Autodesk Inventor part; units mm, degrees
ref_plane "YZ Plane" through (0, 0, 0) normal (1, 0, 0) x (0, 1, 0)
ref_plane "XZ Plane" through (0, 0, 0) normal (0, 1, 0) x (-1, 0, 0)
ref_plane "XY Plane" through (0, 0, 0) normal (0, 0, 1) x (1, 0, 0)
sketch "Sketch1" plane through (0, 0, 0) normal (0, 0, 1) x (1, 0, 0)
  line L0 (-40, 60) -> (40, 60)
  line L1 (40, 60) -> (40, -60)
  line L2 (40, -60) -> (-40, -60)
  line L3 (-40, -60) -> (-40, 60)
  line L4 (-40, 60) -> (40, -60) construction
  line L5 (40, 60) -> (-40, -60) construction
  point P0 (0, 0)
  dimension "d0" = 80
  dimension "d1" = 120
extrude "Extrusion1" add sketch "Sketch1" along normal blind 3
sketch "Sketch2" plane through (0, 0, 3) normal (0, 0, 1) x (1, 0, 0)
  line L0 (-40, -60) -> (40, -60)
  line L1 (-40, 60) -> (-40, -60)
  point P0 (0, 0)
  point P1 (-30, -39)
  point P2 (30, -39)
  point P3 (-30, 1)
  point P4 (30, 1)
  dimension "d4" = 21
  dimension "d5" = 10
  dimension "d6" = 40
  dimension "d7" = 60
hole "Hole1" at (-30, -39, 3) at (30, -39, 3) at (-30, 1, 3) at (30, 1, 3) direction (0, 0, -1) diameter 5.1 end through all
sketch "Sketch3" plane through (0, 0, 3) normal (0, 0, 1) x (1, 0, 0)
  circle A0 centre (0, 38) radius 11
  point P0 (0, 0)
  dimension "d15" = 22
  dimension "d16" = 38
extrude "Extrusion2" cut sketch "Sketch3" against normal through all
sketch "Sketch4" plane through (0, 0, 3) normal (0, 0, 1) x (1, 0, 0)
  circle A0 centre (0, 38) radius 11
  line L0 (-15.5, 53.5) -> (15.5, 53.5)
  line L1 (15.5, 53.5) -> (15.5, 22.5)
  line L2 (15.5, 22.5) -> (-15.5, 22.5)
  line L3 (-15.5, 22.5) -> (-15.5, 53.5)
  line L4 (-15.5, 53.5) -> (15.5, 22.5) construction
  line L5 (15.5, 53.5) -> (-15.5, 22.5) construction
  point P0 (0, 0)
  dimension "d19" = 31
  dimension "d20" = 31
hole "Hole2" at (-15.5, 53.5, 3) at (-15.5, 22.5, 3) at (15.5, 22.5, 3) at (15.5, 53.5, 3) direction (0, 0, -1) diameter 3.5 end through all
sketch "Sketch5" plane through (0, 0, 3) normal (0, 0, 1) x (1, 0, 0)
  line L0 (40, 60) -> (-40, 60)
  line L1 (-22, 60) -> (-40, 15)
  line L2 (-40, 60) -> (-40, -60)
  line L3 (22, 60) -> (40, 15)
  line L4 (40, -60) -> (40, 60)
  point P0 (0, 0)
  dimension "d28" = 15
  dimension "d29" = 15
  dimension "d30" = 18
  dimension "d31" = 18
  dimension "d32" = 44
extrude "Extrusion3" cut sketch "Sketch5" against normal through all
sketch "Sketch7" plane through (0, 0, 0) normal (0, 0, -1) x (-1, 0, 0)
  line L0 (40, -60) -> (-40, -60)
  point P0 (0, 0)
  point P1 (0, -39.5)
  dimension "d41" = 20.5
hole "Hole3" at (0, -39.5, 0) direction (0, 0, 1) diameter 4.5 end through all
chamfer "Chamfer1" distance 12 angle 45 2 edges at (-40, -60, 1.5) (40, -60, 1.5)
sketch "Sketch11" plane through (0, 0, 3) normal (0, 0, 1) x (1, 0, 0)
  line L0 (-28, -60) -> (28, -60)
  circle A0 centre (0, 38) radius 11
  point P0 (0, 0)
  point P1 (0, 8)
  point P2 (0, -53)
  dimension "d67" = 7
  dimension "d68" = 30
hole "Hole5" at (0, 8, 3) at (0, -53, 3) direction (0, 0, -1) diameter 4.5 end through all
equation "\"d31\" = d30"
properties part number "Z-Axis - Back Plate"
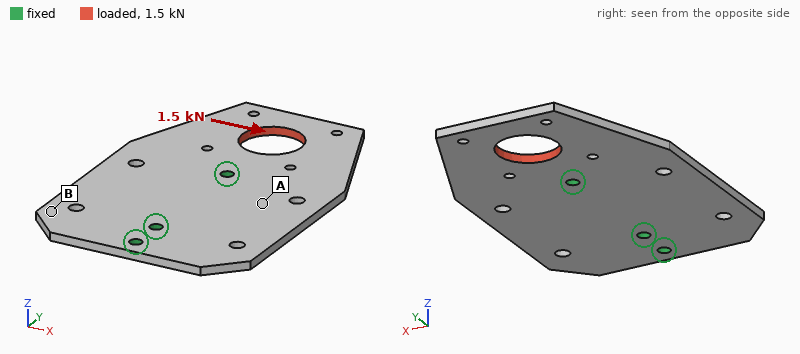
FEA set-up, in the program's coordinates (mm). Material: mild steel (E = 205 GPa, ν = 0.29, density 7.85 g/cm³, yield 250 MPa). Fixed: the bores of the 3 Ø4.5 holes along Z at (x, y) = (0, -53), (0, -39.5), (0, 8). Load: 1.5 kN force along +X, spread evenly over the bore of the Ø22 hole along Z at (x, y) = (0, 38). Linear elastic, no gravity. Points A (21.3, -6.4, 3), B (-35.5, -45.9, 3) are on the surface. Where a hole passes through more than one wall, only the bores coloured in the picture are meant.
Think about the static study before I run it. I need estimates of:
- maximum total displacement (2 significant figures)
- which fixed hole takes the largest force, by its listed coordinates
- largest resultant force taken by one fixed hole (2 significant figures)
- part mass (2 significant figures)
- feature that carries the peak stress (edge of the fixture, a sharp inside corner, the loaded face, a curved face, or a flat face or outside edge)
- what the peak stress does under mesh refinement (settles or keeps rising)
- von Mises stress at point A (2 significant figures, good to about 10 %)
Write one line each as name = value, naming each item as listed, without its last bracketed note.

maximum total displacement = 14 µm
which fixed hole takes the largest force, by its listed coordinates = (0, 8)
largest resultant force taken by one fixed hole = 2.2 kN
part mass = 190 g
feature that carries the peak stress = edge of the fixture
what the peak stress does under mesh refinement = keeps rising
von Mises stress at point A = 8.8 MPa
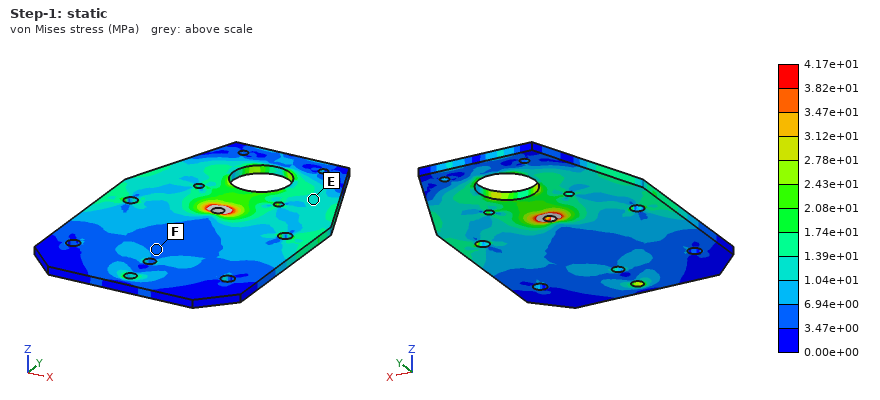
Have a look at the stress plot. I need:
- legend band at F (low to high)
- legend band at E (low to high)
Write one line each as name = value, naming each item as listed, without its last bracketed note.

legend band at F = 3.47e+00 to 6.94e+00 MPa
legend band at E = 1.04e+01 to 1.39e+01 MPa
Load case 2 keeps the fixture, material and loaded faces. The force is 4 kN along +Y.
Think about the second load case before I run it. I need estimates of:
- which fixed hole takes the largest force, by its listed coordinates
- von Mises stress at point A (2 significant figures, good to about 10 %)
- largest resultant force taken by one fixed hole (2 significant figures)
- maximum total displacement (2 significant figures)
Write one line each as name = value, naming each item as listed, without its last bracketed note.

which fixed hole takes the largest force, by its listed coordinates = (0, 8)
von Mises stress at point A = 12 MPa
largest resultant force taken by one fixed hole = 2.7 kN
maximum total displacement = 12 µm
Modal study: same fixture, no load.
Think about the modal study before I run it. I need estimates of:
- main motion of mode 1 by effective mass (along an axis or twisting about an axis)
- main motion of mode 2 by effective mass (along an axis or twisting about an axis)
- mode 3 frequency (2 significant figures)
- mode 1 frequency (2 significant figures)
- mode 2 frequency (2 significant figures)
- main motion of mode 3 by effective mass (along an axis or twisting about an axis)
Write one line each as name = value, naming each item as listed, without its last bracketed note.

main motion of mode 1 by effective mass = along Z
main motion of mode 2 by effective mass = twisting about Y
mode 3 frequency = 1700 Hz
mode 1 frequency = 940 Hz
mode 2 frequency = 1200 Hz
main motion of mode 3 by effective mass = along Z
